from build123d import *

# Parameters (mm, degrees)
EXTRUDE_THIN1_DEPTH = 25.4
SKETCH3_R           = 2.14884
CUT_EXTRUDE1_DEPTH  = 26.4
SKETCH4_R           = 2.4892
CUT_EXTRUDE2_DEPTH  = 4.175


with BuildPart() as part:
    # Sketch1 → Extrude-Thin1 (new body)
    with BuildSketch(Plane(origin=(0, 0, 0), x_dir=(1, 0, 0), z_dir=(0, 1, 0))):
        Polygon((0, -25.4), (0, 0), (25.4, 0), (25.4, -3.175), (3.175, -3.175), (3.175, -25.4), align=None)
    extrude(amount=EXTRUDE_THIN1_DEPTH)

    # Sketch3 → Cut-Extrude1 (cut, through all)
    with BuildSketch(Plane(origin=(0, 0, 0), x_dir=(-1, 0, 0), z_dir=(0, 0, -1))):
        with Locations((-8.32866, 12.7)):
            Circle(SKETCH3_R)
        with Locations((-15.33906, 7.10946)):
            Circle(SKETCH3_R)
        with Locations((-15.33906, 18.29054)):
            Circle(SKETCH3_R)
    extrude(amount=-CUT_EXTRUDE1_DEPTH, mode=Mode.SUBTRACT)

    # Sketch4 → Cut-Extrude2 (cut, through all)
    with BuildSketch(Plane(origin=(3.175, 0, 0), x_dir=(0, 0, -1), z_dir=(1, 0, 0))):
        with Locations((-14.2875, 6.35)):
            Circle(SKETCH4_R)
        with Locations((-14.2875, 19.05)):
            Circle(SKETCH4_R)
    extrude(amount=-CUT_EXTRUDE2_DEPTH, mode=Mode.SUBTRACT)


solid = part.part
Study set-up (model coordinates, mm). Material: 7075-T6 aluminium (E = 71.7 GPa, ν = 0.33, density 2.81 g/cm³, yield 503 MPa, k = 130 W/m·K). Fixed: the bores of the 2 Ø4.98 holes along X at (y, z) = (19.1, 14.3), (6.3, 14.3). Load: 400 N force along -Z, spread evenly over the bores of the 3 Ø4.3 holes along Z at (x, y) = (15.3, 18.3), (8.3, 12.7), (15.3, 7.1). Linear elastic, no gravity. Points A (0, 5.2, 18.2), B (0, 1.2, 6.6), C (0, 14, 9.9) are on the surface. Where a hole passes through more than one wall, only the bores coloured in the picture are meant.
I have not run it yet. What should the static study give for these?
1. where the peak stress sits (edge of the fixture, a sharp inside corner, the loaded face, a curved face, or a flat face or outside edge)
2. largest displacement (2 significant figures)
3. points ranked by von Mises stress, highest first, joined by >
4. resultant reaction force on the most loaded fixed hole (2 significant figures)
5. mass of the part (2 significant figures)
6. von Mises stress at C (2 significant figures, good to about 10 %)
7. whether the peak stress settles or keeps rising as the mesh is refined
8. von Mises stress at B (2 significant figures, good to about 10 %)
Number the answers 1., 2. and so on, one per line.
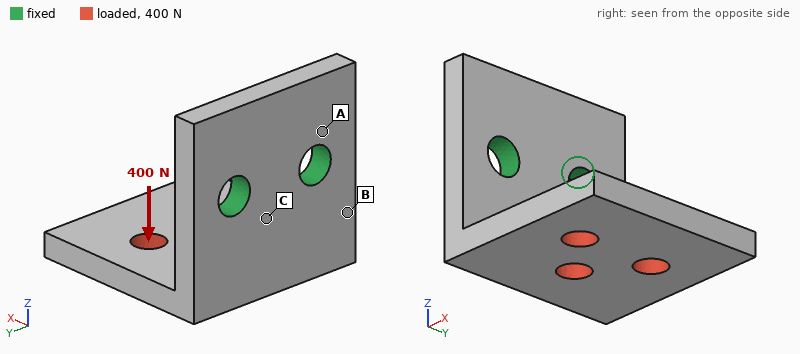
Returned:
1. edge of the fixture
2. 0.34 mm
3. B > C > A
4. 210 N
5. 10 g
6. 79 MPa
7. keeps rising
8. 100 MPa
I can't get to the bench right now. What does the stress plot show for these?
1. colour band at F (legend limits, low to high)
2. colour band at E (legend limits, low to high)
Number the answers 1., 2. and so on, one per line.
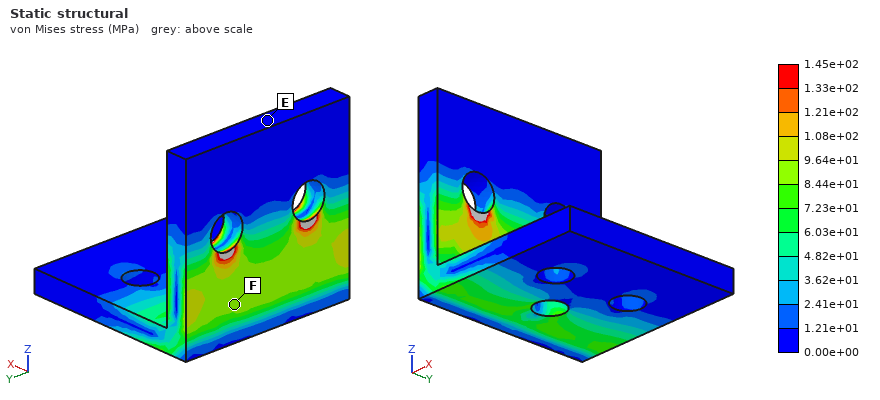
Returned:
1. 8.44e+01 to 9.64e+01 MPa
2. 0.00e+00 to 1.21e+01 MPa
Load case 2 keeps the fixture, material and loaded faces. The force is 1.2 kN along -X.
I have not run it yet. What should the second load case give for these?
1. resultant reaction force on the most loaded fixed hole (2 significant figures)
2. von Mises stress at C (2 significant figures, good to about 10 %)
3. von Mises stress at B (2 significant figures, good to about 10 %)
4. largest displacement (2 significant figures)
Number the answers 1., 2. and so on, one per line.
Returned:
1. 600 N
2. 170 MPa
3. 140 MPa
4. 0.38 mm
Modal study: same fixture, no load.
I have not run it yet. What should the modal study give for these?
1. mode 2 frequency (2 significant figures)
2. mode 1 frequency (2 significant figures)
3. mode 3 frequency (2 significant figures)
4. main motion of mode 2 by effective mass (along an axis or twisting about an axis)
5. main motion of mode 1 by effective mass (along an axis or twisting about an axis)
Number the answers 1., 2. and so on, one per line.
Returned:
1. 5300 Hz
2. 2700 Hz
3. 9200 Hz
4. along Y
5. along Z
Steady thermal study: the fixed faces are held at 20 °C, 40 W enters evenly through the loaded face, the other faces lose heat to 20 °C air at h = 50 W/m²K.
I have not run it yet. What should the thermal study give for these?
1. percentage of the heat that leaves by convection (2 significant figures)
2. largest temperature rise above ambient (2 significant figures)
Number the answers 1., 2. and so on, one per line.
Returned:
1. 13 %
2. 83 K
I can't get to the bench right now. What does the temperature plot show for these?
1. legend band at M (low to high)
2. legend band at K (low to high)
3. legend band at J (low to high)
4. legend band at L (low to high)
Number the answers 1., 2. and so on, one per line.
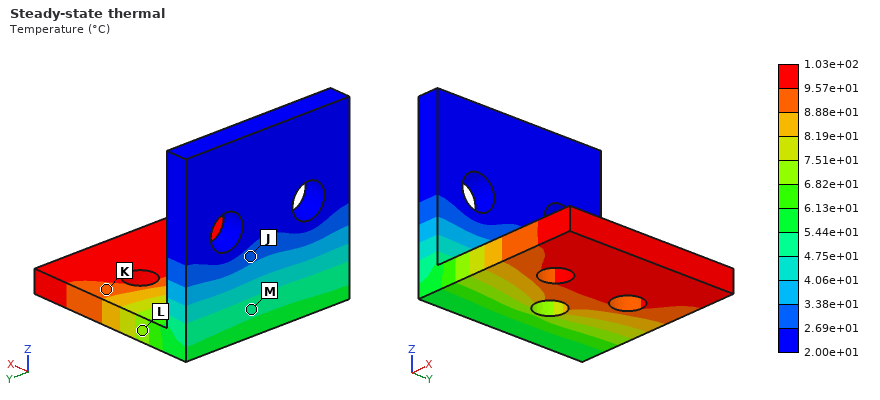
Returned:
1. 4.75e+01 to 5.44e+01 °C
2. 8.88e+01 to 9.57e+01 °C
3. 2.69e+01 to 3.38e+01 °C
4. 6.82e+01 to 7.51e+01 °C
